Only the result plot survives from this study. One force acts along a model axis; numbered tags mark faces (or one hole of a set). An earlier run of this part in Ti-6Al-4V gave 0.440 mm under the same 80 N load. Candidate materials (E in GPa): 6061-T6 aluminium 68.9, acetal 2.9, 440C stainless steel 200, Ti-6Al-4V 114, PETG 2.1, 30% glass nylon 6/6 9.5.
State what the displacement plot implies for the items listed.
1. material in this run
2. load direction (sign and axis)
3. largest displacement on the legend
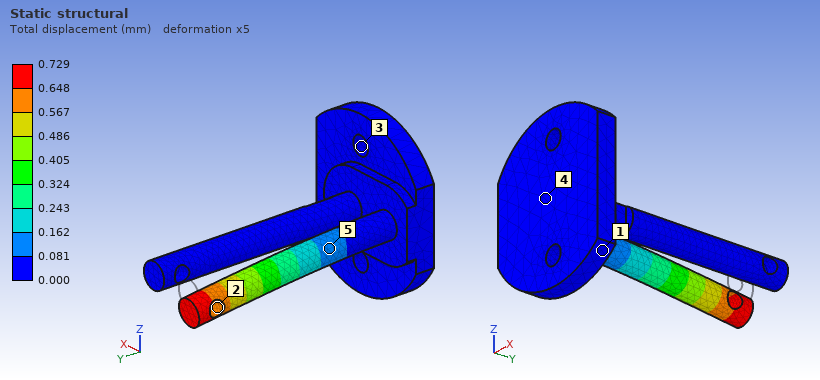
6061-T6 aluminium
-Z
0.729 mm
